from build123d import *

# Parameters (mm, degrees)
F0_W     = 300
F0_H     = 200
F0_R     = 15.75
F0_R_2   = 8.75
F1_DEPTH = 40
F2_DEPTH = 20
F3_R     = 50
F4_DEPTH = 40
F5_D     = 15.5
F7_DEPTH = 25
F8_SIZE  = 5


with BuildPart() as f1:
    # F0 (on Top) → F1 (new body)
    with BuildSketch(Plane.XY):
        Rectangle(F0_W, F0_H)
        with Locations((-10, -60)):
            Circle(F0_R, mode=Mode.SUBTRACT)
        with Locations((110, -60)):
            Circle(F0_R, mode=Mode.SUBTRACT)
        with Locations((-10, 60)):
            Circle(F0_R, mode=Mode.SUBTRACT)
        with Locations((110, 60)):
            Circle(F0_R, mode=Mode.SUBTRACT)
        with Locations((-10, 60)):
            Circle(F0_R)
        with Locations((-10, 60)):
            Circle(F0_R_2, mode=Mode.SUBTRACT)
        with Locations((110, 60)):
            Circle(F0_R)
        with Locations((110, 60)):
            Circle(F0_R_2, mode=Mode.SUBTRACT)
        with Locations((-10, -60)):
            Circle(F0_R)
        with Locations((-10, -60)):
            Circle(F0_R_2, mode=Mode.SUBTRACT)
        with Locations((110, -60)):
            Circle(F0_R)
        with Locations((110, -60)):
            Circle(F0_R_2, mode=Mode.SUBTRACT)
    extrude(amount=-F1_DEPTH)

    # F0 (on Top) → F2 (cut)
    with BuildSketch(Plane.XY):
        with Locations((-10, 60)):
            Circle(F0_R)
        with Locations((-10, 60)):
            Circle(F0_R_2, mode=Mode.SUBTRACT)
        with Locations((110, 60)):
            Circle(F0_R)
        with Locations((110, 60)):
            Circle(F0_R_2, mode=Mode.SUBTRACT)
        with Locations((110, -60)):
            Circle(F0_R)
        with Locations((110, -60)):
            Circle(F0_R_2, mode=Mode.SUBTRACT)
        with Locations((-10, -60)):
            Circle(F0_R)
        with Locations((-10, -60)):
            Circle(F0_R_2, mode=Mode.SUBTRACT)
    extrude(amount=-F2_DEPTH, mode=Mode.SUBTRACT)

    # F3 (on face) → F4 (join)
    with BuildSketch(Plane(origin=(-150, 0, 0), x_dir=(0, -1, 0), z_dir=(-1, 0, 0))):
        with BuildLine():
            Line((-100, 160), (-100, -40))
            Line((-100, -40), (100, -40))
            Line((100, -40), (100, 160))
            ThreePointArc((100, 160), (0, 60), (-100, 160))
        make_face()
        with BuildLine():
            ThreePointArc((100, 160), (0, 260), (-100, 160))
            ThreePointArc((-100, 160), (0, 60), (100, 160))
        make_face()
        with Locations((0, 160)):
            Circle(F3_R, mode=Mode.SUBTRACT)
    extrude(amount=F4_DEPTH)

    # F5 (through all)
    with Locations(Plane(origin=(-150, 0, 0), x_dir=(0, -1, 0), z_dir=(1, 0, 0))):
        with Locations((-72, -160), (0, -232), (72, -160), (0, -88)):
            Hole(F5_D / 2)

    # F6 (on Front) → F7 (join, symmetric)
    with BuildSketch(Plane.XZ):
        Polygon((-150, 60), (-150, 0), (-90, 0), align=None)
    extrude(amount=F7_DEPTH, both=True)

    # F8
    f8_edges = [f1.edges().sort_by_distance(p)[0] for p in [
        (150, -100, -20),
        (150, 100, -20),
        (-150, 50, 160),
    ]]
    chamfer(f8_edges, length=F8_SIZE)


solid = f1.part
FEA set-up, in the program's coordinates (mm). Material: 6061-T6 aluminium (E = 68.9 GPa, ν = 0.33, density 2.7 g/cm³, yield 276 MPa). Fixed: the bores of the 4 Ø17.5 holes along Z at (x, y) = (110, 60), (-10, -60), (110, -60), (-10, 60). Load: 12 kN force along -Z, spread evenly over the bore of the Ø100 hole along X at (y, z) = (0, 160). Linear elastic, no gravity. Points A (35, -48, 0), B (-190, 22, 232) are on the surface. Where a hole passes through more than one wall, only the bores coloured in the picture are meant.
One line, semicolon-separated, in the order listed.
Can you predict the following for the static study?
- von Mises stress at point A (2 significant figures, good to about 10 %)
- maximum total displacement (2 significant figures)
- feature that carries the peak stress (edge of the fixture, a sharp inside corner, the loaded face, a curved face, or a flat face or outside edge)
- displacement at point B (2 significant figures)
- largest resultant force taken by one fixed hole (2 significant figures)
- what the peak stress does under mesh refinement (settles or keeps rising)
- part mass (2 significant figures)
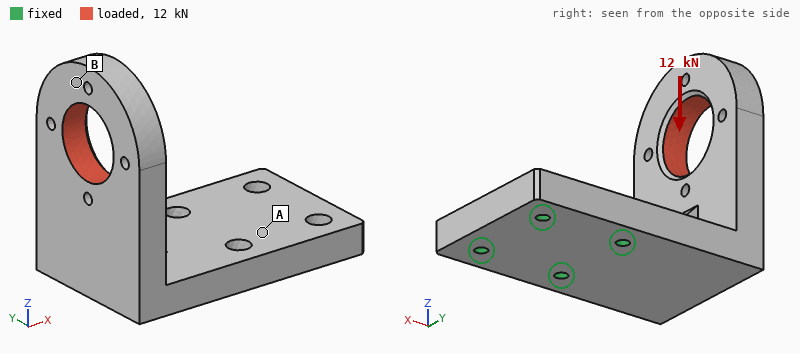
12 MPa; 0.87 mm; edge of the fixture; 0.80 mm; 15 kN; keeps rising; 12 kg
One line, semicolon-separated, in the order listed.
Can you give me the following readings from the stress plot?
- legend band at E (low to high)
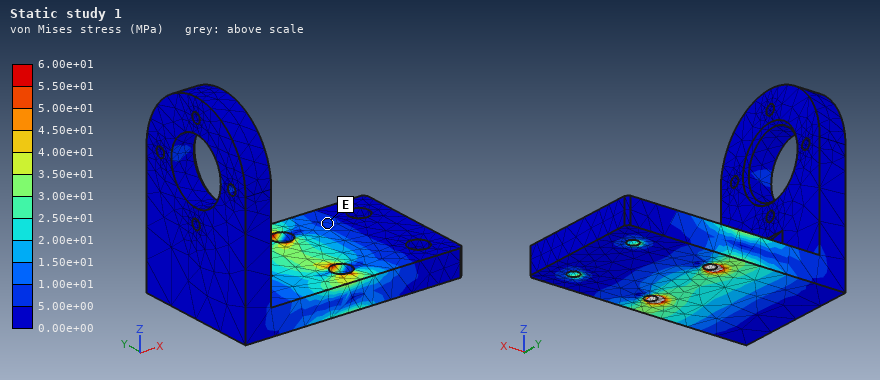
5.00e+00 to 1.00e+01 MPa
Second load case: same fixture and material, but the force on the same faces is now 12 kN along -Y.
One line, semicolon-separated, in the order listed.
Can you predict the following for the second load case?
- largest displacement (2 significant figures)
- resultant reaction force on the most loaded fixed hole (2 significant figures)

0.63 mm; 26 kN
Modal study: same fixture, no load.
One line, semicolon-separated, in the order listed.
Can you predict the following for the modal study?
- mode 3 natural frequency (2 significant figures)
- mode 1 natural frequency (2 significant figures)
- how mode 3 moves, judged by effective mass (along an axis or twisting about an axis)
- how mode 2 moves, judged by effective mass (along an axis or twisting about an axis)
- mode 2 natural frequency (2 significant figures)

790 Hz; 260 Hz; along Z; along Y; 460 Hz
